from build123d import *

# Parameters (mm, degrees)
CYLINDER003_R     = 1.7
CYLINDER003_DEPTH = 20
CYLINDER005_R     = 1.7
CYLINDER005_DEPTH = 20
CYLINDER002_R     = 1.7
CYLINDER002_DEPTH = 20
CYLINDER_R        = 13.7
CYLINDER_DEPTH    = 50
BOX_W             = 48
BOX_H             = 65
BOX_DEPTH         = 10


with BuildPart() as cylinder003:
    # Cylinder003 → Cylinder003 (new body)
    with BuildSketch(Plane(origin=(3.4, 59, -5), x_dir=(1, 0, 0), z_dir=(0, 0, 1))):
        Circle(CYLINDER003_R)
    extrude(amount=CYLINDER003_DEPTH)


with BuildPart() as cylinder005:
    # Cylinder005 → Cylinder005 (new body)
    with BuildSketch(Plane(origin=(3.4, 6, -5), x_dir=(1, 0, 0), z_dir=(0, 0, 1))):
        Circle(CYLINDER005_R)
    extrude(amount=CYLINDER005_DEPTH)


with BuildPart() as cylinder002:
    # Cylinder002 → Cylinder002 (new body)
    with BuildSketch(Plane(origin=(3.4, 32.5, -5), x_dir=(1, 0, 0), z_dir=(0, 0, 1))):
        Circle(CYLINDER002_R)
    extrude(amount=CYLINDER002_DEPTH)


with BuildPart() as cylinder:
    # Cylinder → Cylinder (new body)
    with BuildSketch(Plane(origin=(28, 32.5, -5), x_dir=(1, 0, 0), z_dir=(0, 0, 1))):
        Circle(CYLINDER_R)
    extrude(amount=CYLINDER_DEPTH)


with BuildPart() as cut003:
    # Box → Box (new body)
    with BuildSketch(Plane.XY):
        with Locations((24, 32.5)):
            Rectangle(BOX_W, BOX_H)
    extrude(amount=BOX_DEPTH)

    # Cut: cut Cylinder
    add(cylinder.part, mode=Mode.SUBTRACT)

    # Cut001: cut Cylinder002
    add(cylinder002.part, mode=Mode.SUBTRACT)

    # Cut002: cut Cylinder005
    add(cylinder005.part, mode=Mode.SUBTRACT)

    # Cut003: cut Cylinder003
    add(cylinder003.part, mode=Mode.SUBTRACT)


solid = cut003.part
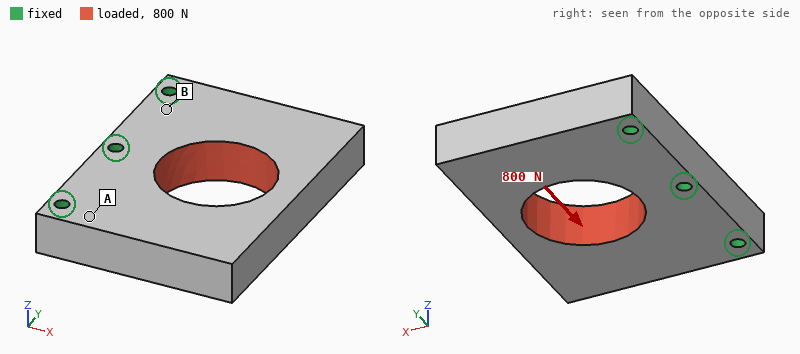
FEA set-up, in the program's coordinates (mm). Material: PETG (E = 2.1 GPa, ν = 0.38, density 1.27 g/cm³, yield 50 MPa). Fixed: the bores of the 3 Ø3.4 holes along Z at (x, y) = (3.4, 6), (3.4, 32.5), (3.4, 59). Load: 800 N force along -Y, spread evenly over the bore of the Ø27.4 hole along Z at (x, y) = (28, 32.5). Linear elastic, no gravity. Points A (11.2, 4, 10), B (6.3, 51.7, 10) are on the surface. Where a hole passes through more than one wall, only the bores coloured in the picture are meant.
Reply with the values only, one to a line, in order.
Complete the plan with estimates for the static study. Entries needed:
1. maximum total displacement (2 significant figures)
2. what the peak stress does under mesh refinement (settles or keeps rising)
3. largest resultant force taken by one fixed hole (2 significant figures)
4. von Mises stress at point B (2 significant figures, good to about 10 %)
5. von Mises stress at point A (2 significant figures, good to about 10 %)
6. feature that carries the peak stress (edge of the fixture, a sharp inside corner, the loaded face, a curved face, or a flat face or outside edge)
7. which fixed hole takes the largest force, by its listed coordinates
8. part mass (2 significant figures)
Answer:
0.19 mm
keeps rising
490 N
1.2 MPa
3.0 MPa
edge of the fixture
(3.4, 32.5)
32 g
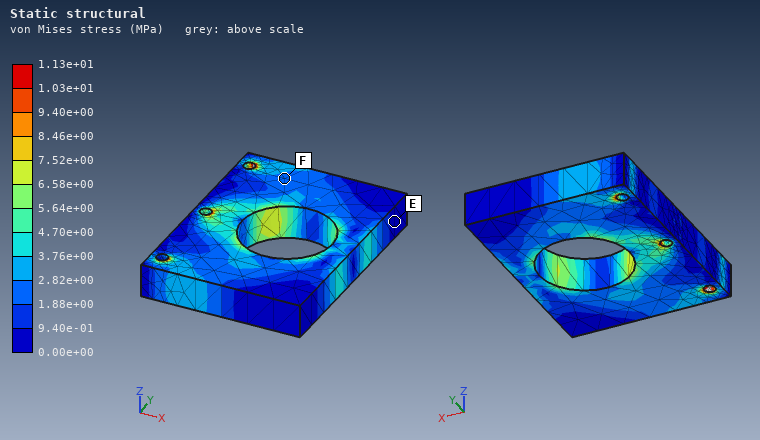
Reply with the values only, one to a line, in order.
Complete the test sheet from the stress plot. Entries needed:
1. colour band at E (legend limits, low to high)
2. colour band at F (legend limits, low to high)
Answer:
0.00e+00 to 9.40e-01 MPa
1.88e+00 to 2.82e+00 MPa
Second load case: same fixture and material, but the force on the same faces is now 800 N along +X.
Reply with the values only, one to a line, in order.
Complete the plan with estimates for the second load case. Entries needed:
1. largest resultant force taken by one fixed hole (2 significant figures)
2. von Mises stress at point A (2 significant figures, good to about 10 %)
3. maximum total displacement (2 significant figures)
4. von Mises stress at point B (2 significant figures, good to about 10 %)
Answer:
290 N
1.7 MPa
77 µm
1.5 MPa
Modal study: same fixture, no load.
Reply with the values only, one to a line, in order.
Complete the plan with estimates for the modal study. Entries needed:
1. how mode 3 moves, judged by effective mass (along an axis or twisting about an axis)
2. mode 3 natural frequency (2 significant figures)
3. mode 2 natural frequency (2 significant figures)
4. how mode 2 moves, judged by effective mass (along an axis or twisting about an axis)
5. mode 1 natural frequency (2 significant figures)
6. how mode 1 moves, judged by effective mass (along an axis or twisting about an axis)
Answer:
along Y
2400 Hz
1400 Hz
twisting about X
850 Hz
along Z
